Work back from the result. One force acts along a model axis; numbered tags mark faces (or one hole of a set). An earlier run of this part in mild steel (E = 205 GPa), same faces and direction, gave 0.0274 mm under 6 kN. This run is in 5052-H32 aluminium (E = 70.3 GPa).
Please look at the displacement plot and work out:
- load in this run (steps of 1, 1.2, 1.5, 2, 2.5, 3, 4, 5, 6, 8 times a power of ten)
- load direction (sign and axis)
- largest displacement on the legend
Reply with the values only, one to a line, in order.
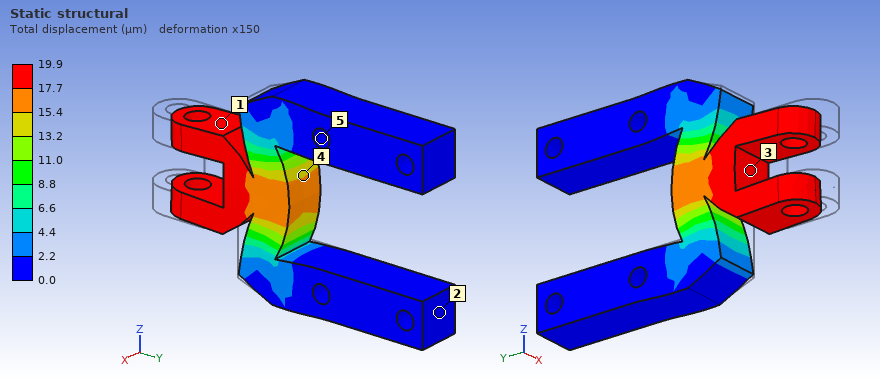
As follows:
1.5 kN
+Y
19.9 µm
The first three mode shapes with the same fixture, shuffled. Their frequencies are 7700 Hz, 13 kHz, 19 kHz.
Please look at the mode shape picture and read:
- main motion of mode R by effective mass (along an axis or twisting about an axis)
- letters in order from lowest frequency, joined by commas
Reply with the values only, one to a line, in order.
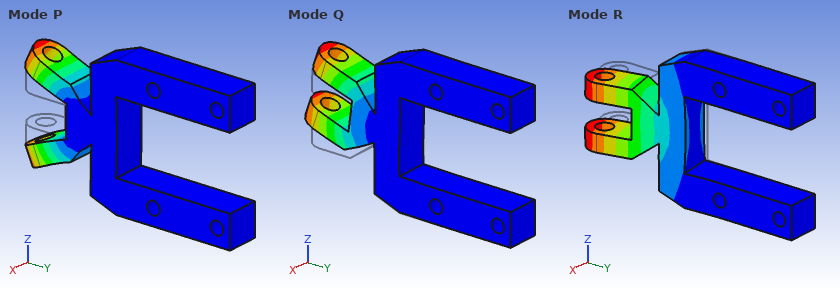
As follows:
along X
R, Q, P
